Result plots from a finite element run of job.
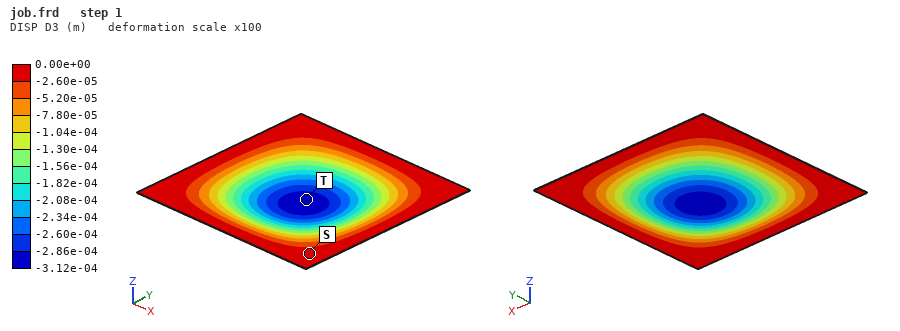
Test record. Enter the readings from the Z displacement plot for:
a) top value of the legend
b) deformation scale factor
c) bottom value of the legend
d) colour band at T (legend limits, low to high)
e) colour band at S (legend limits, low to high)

0.00e+00 m
100
-3.12e-04 m
-3.12e-04 to -2.86e-04 m
-2.60e-05 to 0.00e+00 m
